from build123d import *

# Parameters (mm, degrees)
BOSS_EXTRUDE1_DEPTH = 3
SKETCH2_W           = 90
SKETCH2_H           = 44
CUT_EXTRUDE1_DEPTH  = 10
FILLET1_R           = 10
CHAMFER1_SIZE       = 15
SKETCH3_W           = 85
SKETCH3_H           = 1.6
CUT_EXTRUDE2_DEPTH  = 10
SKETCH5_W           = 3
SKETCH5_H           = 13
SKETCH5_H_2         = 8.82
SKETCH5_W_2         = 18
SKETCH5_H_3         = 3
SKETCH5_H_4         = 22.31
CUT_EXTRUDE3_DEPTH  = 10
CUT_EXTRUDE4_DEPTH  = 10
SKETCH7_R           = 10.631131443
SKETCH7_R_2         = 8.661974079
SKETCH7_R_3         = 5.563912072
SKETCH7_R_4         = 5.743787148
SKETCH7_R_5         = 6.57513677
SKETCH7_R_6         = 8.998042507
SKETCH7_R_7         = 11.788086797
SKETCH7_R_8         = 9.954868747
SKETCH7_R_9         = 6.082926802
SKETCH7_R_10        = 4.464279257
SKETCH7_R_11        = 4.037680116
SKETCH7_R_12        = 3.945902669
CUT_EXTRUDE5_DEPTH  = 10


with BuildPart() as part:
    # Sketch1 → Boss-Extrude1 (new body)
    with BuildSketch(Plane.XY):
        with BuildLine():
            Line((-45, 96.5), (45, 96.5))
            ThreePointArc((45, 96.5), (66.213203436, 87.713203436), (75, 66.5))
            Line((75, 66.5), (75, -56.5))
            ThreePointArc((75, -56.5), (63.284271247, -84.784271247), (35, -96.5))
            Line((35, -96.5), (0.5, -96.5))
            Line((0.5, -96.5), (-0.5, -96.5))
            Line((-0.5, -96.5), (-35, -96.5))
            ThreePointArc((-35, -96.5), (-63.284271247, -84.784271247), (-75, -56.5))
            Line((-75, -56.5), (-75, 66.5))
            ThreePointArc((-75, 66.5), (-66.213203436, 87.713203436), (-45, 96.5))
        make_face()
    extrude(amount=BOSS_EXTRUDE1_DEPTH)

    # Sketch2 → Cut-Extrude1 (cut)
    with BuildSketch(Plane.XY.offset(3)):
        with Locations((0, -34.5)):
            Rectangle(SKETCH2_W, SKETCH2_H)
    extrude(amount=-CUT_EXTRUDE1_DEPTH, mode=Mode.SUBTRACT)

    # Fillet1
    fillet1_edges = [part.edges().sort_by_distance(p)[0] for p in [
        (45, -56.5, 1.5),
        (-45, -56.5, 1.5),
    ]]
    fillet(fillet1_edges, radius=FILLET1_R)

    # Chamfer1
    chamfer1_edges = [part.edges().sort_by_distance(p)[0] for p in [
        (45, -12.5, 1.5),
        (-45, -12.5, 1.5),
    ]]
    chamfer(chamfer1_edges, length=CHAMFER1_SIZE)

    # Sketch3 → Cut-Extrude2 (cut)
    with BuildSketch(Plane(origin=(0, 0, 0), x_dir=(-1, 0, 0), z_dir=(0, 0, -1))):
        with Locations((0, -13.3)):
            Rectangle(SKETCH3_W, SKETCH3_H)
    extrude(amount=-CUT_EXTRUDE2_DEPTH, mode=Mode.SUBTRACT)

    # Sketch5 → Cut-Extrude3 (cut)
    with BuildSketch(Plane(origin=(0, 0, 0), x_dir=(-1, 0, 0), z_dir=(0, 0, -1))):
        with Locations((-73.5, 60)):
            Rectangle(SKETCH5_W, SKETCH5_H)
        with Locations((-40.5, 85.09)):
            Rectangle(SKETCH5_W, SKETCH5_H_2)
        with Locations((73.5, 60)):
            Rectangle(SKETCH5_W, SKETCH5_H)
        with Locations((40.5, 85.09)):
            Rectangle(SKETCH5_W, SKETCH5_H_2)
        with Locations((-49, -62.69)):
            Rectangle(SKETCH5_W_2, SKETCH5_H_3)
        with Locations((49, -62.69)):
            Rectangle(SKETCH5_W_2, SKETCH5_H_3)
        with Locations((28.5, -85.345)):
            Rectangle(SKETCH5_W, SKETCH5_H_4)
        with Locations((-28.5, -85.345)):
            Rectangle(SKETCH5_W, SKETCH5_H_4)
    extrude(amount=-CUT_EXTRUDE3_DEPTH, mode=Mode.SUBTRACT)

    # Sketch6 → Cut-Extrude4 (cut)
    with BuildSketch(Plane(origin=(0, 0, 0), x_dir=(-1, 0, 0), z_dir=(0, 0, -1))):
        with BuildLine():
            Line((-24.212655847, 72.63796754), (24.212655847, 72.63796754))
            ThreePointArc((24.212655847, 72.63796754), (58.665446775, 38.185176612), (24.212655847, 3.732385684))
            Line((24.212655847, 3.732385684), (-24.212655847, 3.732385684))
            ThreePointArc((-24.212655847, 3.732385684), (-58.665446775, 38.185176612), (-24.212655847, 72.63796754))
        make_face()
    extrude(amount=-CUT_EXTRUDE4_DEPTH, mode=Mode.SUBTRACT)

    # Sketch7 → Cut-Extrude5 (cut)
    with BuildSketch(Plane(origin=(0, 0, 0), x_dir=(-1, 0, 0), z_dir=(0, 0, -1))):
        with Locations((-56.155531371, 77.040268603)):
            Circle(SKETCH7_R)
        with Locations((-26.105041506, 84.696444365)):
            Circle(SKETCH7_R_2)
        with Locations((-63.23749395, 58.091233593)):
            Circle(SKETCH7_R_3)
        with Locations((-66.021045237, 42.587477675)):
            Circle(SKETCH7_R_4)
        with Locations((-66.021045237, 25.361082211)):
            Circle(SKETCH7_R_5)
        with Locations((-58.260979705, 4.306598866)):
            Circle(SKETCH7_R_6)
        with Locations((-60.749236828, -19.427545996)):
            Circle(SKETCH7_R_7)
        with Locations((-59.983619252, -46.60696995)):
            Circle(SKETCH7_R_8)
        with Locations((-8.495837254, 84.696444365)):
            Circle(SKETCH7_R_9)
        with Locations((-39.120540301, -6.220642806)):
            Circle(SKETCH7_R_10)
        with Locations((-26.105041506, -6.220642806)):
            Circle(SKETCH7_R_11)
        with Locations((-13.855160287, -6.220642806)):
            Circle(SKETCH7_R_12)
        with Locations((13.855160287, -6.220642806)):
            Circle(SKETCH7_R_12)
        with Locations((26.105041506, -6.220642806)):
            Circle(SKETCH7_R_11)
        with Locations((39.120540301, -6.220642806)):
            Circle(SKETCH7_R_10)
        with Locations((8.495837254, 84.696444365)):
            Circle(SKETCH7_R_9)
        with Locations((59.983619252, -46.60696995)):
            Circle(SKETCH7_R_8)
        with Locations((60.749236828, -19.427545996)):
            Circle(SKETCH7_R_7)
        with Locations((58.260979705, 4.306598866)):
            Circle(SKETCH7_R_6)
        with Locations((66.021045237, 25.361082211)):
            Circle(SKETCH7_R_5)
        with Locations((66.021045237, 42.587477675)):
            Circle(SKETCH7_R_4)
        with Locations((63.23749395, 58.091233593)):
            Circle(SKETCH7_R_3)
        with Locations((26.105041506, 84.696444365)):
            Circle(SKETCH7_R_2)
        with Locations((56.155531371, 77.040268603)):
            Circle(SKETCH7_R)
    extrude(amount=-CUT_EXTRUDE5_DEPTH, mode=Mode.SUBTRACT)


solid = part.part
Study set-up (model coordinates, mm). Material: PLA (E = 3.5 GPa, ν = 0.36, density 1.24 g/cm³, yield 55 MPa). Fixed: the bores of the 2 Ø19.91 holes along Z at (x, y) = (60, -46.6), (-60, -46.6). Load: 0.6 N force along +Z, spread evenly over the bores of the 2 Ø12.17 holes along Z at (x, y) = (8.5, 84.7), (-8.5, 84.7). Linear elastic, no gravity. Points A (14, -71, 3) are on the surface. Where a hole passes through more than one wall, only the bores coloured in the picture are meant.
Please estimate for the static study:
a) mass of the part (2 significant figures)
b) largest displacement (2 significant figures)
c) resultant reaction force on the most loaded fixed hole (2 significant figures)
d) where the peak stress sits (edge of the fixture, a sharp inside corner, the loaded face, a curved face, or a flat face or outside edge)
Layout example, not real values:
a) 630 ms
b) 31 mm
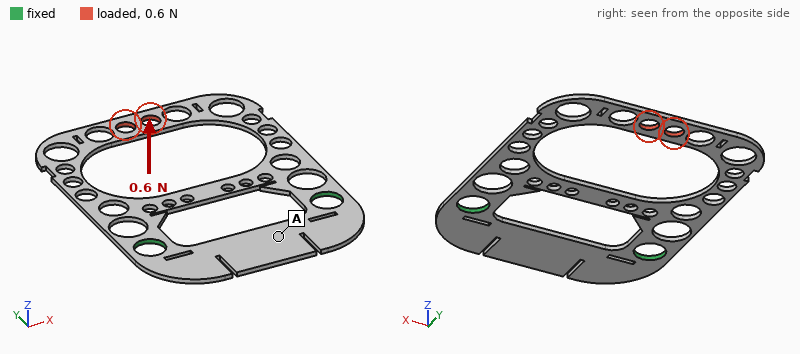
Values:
a) 46 g
b) 2.4 mm
c) 0.30 N
d) a curved face
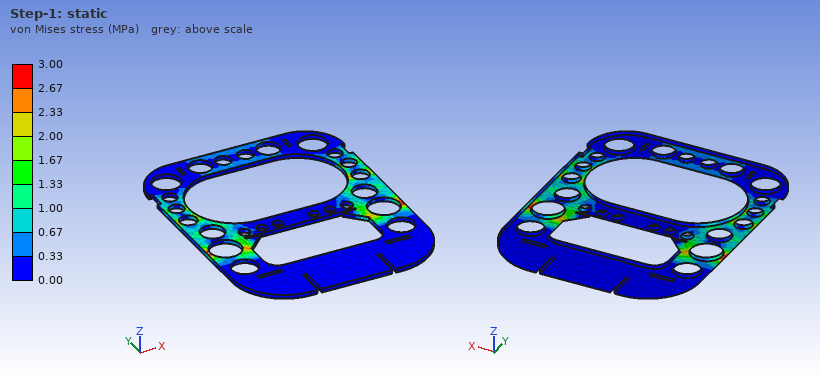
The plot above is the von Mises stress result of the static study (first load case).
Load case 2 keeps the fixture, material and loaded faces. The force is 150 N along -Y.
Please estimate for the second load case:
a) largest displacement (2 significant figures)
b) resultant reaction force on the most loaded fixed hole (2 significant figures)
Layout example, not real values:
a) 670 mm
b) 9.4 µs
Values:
a) 0.88 mm
b) 75 N
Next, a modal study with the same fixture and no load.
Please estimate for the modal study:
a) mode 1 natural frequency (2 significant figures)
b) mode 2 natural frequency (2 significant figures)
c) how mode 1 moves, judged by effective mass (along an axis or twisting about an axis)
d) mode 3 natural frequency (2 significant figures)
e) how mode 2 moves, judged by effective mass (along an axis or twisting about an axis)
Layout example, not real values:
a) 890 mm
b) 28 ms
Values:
a) 29 Hz
b) 78 Hz
c) along Z
d) 180 Hz
e) twisting about Y
